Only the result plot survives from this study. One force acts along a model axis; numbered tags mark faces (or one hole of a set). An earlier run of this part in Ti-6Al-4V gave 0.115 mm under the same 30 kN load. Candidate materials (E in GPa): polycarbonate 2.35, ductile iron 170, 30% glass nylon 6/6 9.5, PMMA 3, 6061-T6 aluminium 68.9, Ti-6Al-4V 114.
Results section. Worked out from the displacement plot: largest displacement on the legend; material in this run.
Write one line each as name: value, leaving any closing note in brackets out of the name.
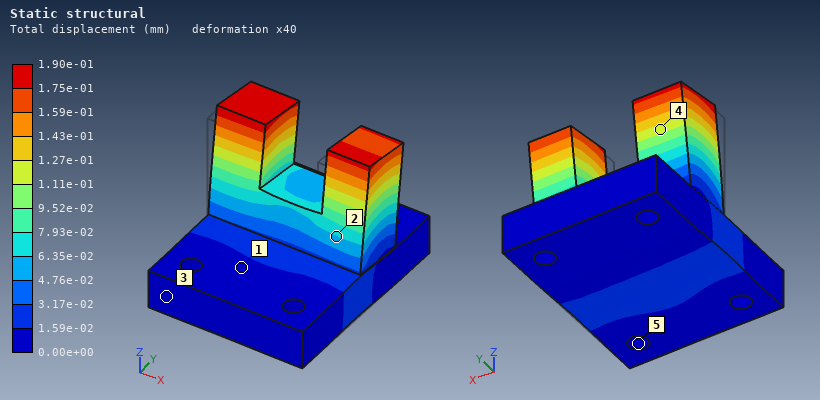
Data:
largest displacement on the legend: 1.90e-01 mm
material in this run: 6061-T6 aluminium
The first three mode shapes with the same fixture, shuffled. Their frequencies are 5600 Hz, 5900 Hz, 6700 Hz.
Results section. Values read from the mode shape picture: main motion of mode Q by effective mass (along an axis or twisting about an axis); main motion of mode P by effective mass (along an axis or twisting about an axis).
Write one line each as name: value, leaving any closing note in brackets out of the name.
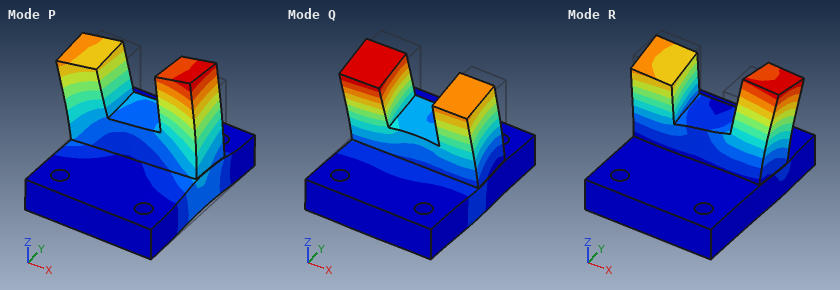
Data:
main motion of mode Q by effective mass: along Y
main motion of mode P by effective mass: along X
